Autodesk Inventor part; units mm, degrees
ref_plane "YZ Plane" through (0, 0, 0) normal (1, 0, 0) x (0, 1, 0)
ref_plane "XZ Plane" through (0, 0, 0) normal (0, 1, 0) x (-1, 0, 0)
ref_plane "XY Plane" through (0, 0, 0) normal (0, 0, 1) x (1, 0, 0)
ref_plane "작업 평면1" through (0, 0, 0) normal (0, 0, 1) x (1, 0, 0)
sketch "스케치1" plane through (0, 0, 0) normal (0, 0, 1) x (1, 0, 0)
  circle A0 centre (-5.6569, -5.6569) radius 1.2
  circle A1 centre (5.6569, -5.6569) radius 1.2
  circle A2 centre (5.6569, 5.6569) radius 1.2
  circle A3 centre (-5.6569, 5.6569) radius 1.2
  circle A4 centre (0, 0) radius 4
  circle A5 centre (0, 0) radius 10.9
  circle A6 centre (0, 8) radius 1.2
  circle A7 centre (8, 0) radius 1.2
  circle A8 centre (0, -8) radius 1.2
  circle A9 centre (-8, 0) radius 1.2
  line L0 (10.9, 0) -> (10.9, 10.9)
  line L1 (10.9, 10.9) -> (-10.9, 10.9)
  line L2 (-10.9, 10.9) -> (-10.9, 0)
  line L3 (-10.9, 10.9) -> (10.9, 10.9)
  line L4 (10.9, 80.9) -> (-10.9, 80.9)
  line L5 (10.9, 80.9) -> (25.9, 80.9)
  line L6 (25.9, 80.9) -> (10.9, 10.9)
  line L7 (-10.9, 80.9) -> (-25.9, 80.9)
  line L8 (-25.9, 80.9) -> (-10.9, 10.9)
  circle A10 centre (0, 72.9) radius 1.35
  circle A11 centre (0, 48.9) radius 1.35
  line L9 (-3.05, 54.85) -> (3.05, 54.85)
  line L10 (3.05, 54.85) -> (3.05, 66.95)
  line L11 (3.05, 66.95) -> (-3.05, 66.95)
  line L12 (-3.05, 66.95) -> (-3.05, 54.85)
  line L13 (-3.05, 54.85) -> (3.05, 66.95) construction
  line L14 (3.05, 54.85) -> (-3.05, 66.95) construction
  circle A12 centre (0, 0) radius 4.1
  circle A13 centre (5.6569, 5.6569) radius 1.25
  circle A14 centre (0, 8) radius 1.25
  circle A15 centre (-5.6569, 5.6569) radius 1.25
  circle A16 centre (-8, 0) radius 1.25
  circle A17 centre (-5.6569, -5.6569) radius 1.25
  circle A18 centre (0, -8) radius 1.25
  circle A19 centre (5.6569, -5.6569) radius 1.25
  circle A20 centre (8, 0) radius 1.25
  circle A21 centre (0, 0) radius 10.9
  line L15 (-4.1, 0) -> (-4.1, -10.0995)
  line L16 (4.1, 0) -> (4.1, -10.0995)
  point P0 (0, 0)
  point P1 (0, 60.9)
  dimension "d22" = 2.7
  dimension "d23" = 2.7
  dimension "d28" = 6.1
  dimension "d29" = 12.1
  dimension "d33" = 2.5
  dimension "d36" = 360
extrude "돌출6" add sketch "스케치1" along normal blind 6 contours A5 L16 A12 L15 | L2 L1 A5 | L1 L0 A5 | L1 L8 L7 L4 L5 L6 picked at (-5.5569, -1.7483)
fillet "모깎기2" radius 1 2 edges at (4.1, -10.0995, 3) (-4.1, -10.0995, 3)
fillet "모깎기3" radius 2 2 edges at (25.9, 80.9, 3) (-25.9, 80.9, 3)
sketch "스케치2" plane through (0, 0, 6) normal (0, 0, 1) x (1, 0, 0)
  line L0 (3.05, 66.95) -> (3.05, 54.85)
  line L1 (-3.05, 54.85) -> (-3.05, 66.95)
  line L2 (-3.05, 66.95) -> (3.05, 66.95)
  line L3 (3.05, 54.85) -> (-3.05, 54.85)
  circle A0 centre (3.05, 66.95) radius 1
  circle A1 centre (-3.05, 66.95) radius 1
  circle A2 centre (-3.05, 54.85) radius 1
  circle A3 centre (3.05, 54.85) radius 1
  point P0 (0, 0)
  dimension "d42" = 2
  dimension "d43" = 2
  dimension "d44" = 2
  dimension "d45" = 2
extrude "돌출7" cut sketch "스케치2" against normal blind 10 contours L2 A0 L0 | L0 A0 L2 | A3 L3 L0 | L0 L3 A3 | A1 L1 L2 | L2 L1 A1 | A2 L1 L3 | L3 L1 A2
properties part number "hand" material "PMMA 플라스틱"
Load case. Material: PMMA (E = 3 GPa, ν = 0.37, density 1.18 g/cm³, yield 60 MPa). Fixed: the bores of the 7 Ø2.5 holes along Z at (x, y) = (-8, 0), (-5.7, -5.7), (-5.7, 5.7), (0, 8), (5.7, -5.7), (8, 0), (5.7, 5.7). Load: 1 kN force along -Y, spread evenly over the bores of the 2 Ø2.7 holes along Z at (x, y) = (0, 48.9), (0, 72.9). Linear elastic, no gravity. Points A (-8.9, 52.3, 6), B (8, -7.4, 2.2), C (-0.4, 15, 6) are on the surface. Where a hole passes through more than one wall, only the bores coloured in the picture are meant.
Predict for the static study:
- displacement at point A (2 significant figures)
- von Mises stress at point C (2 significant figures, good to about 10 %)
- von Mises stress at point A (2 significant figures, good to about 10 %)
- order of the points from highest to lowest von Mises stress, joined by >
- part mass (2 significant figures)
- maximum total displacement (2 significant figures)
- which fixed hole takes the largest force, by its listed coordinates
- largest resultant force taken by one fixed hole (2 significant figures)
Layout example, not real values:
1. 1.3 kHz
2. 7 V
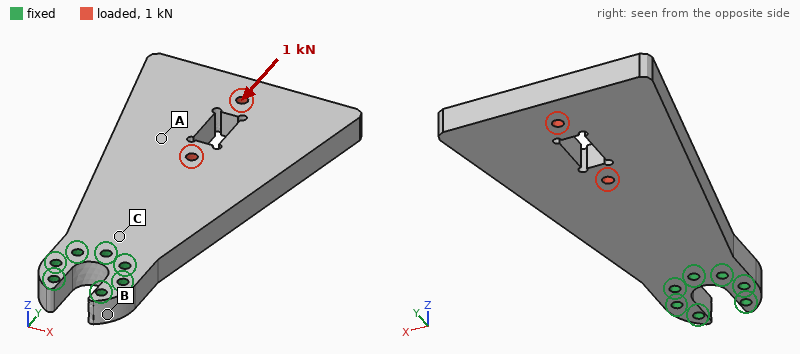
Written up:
1. 0.089 mm
2. 7.9 MPa
3. 4.5 MPa
4. C > A > B
5. 19 g
6. 0.14 mm
7. (0, 8)
8. 320 N
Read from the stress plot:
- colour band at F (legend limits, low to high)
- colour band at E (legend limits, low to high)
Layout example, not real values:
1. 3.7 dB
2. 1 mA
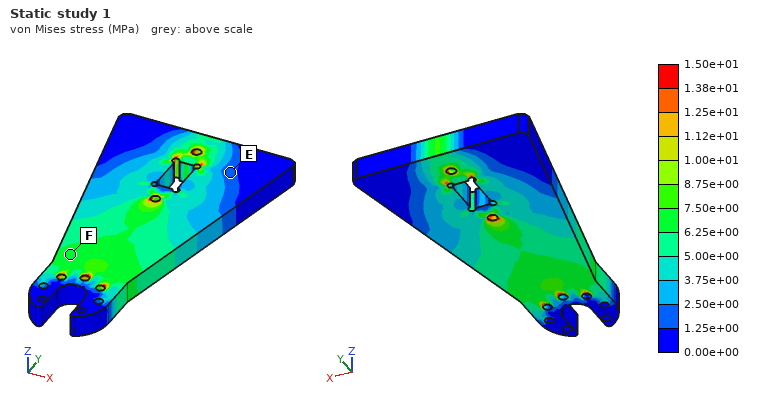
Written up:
1. 6.25e+00 to 7.50e+00 MPa
2. 1.25e+00 to 2.50e+00 MPa
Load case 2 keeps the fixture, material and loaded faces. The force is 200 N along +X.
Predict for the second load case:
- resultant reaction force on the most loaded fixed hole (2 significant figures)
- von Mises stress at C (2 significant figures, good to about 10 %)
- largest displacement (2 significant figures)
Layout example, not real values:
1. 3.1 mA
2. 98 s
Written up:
1. 510 N
2. 6.5 MPa
3. 1.0 mm
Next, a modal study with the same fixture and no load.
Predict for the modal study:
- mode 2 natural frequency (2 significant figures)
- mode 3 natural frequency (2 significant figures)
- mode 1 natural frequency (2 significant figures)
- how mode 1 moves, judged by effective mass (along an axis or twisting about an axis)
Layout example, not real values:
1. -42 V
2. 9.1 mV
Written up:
1. 710 Hz
2. 720 Hz
3. 220 Hz
4. along Z
